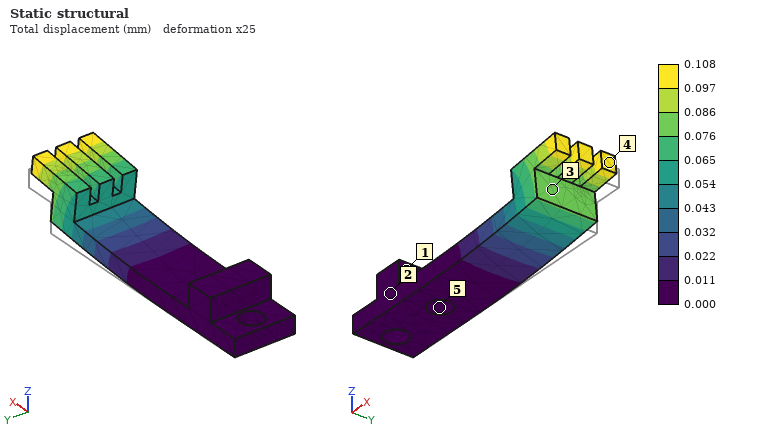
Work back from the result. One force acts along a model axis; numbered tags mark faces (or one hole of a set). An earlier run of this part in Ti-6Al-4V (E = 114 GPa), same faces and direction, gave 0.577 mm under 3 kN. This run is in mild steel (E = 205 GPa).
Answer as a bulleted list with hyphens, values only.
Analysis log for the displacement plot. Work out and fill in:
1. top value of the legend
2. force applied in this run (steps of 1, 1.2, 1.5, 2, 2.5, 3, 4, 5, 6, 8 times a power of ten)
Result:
- 0.108 mm
- 1 kN
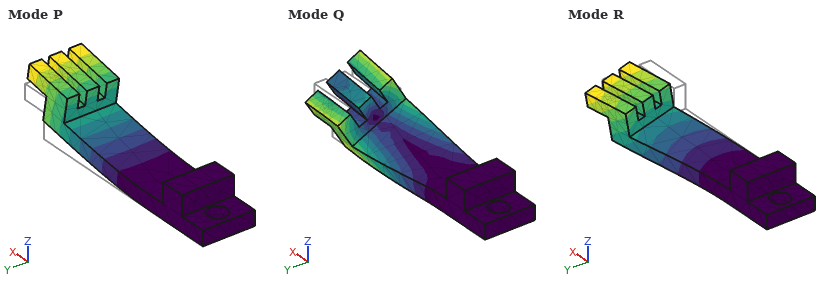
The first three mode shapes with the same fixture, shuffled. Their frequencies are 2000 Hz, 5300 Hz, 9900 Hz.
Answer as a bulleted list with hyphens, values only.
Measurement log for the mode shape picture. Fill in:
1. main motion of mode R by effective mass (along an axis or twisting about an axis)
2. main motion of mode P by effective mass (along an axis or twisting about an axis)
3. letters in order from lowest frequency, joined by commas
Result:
- along Y
- along Z
- P, R, Q
